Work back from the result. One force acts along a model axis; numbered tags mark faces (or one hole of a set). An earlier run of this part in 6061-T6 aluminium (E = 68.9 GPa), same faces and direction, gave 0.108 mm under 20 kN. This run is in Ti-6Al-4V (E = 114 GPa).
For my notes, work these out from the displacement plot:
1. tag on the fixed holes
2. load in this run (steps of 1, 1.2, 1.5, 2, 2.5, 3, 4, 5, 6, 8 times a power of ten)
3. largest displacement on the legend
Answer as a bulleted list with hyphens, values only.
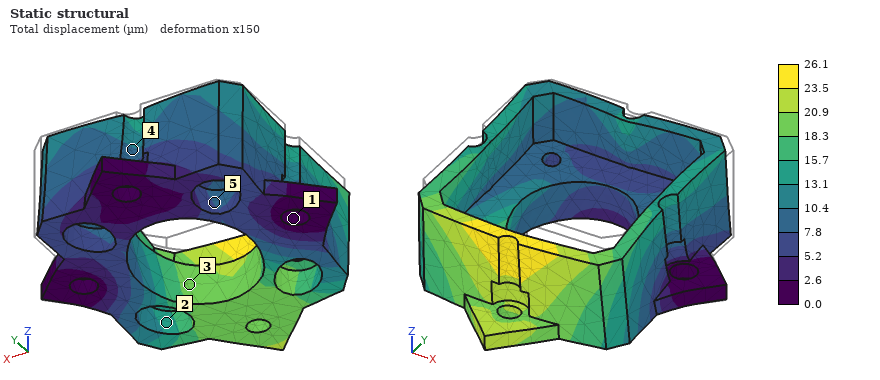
- 1
- 8 kN
- 26.1 µm
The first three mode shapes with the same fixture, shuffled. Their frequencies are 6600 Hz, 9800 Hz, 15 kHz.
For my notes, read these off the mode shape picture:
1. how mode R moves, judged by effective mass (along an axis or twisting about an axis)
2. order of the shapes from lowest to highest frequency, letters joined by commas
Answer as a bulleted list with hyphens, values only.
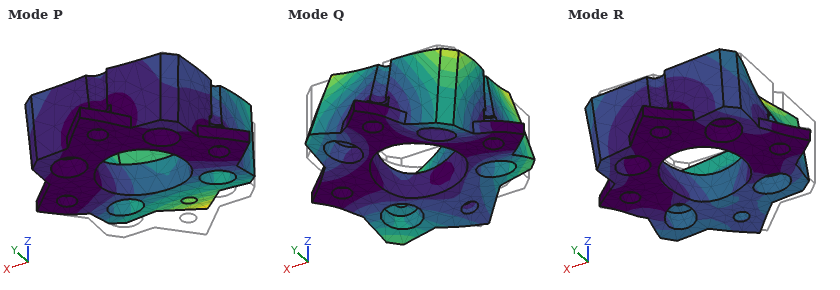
- along X
- P, Q, R
